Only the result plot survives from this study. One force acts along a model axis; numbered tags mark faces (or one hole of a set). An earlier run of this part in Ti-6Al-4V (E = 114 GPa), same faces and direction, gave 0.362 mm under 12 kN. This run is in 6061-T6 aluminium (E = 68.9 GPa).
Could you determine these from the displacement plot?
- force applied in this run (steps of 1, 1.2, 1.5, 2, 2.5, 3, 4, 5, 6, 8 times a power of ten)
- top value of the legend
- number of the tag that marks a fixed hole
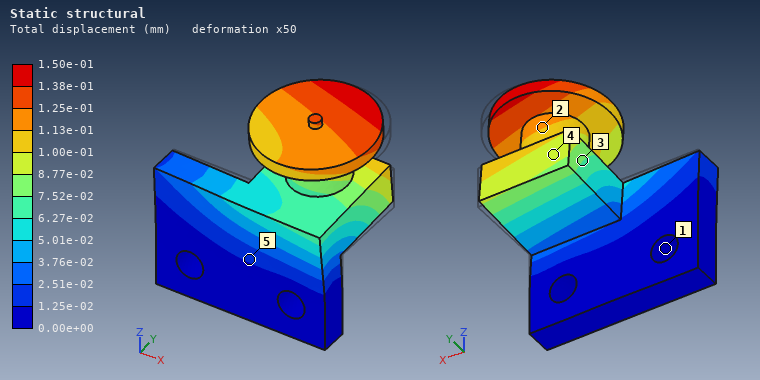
3 kN
1.50e-01 mm
1
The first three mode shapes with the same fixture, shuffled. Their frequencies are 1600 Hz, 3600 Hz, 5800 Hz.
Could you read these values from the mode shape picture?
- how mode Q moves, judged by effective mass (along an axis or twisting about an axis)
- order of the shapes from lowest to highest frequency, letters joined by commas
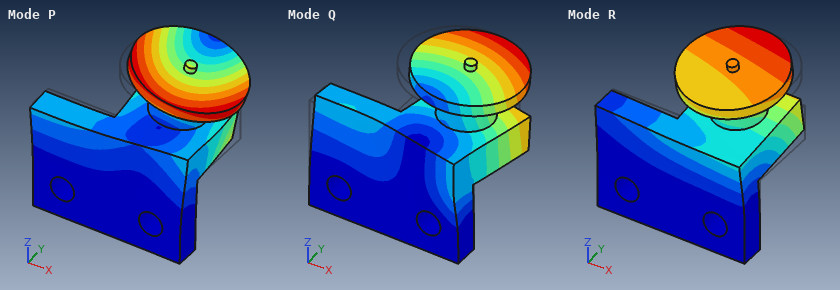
along X
R, Q, P
